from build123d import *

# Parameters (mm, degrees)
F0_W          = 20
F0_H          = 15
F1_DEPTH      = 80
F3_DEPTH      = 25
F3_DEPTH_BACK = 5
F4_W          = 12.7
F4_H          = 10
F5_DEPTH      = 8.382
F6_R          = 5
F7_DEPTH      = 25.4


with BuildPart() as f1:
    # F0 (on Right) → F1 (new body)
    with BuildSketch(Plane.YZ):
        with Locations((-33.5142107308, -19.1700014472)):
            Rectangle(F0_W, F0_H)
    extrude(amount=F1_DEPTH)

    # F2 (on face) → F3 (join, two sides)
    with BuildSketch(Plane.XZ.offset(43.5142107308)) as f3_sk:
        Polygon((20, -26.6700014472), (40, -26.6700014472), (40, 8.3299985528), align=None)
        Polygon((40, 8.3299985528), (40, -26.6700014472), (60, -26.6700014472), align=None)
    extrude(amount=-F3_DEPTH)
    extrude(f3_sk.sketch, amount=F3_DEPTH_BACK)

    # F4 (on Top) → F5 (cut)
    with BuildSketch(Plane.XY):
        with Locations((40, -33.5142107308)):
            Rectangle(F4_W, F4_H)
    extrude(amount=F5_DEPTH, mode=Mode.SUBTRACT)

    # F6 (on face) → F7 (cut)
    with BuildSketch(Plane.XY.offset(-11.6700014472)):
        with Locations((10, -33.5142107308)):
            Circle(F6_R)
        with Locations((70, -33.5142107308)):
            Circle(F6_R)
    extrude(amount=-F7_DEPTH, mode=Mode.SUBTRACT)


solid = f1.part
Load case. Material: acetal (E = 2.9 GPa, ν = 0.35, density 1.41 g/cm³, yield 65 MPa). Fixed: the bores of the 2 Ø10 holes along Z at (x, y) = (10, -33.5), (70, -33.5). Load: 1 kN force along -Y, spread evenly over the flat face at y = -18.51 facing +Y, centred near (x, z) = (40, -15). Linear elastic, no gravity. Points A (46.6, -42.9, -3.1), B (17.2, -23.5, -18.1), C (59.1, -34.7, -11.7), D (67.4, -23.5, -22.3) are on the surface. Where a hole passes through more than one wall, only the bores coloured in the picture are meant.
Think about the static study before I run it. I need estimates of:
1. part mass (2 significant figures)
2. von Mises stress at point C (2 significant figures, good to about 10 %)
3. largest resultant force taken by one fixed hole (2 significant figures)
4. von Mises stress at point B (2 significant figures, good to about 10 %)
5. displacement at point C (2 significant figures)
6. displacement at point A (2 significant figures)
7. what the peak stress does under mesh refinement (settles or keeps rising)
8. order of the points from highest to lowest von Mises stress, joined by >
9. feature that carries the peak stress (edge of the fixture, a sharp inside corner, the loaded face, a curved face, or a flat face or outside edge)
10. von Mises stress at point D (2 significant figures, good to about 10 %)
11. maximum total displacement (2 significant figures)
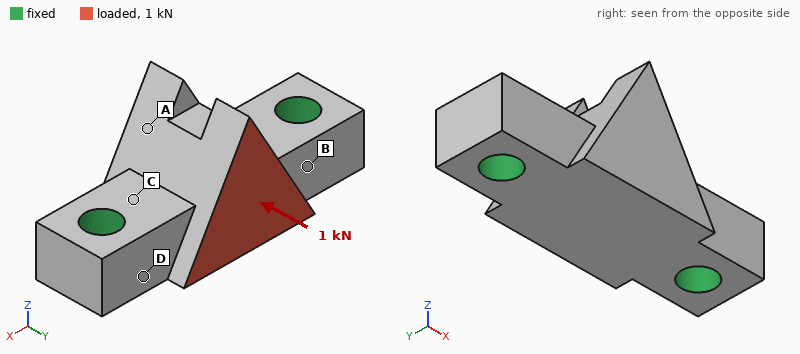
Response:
46 g
6.8 MPa
500 N
3.4 MPa
0.029 mm
0.095 mm
keeps rising
C > B > D > A
edge of the fixture
2.6 MPa
0.16 mm
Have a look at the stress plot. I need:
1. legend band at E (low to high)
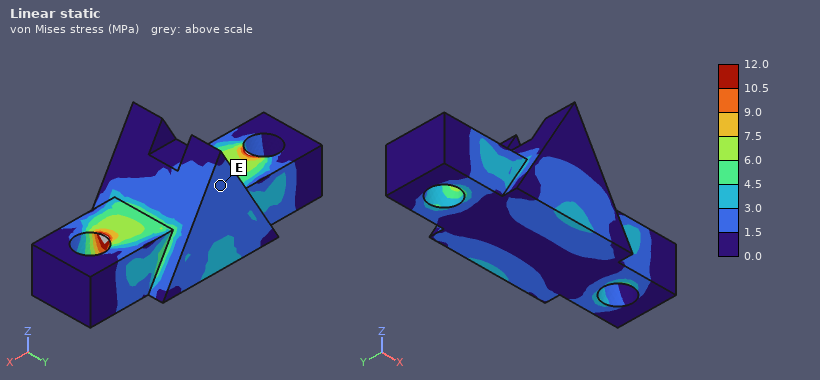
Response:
1.5 to 3.0 MPa
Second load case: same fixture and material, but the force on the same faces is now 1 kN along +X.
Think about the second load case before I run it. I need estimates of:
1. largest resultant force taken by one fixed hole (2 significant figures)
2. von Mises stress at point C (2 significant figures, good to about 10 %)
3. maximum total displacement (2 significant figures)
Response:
580 N
2.3 MPa
79 µm
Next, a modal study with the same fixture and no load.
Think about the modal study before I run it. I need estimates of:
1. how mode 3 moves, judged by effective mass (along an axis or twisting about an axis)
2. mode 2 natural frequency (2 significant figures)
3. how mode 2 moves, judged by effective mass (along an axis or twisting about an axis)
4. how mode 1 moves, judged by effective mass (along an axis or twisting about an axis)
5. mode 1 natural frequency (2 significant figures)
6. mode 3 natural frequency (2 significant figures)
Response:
along Y
4100 Hz
along Z
along Y
2900 Hz
5100 Hz
